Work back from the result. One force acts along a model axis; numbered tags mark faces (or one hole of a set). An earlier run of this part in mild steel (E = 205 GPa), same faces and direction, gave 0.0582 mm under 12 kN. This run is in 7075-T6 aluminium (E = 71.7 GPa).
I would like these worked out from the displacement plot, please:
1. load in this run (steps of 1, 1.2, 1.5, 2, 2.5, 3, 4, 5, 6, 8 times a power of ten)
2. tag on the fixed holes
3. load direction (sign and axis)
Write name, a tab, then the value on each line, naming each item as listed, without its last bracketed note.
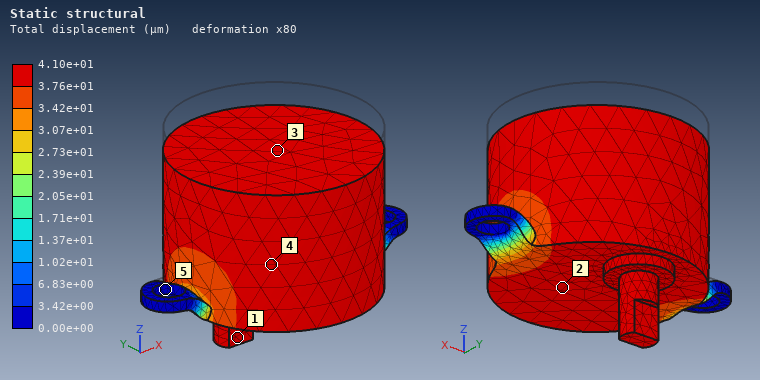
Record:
load in this run	3 kN
tag on the fixed holes	5
load direction	-Z
